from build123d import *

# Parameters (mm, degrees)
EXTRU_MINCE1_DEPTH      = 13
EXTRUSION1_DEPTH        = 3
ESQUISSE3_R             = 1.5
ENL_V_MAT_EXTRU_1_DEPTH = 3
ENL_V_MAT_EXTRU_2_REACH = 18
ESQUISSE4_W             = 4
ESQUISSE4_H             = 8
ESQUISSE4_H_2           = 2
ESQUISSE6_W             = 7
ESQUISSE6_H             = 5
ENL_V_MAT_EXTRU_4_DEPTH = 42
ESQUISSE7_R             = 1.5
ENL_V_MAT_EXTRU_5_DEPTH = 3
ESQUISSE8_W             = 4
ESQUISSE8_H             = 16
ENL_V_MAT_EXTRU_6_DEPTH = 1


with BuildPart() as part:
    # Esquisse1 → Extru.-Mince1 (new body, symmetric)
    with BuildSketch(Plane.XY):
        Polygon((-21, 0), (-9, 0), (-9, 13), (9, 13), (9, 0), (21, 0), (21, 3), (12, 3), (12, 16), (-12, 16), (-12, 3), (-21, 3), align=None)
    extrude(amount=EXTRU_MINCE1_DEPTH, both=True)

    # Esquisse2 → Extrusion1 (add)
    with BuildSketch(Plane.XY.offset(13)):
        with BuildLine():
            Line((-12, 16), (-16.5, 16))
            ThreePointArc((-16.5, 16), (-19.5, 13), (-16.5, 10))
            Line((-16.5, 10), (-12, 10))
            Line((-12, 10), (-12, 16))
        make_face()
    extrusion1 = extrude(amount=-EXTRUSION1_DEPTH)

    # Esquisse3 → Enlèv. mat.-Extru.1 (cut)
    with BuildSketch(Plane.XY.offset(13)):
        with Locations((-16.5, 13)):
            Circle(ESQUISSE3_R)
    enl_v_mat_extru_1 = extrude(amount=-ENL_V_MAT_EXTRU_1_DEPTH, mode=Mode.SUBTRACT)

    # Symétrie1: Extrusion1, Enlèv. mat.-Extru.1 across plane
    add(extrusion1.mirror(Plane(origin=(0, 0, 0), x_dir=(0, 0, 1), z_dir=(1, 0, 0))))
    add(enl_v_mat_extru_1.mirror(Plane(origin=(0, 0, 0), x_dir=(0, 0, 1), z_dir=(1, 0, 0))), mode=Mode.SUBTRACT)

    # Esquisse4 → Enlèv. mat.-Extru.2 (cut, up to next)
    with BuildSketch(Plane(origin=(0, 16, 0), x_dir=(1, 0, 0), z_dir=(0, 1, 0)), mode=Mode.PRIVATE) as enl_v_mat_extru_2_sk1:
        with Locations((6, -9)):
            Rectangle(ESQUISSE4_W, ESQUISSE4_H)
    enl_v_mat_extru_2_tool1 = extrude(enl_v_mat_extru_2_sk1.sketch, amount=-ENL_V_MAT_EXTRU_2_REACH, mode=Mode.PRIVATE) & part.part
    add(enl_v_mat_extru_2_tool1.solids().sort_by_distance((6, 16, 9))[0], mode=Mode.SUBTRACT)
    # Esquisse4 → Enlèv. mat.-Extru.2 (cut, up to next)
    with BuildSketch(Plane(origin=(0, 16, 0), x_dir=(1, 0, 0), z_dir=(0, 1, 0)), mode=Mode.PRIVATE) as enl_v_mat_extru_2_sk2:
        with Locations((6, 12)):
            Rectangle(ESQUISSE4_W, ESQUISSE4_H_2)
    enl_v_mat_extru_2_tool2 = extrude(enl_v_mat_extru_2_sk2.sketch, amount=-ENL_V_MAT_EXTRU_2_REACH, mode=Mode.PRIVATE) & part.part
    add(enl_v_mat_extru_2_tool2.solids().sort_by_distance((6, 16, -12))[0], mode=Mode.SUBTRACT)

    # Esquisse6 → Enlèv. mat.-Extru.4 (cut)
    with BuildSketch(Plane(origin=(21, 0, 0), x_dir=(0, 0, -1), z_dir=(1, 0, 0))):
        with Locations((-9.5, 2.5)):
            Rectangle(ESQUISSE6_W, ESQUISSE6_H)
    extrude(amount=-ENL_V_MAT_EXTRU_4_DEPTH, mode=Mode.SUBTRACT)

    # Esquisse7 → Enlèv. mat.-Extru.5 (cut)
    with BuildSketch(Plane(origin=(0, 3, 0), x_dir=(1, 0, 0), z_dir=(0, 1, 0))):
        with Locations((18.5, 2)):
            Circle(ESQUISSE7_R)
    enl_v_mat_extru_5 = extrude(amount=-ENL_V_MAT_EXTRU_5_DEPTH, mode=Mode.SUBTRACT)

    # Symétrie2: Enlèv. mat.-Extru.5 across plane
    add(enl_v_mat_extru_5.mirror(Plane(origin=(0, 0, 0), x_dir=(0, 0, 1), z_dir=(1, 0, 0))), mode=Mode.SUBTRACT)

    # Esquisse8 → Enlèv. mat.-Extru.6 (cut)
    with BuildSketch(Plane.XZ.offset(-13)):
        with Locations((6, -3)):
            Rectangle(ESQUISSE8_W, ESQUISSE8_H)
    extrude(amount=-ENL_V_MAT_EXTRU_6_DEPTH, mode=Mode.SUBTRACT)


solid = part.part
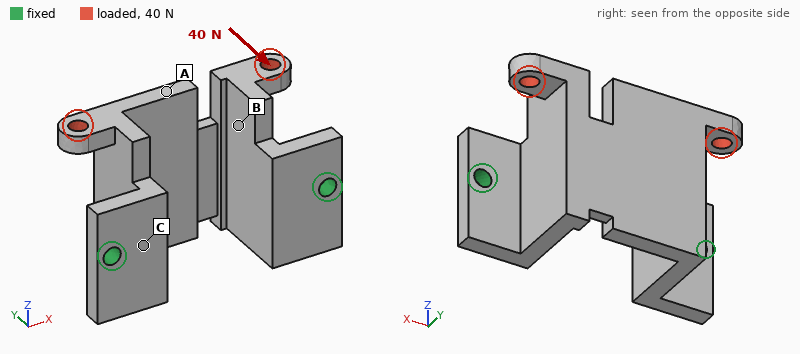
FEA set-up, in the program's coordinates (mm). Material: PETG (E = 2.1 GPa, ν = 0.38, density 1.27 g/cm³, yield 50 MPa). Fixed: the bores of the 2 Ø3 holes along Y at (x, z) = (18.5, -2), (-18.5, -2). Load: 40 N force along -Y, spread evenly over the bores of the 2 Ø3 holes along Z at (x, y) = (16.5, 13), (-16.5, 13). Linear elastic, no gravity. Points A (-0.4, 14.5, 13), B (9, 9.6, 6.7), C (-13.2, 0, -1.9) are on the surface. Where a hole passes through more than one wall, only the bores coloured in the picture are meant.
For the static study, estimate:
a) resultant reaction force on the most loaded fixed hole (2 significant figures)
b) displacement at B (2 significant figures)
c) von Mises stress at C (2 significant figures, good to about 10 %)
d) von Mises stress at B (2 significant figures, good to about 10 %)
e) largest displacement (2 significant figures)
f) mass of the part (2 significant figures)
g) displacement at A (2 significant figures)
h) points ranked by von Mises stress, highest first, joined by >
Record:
21 N
0.21 mm
6.5 MPa
3.8 MPa
0.52 mm
6.0 g
0.33 mm
C > B > A
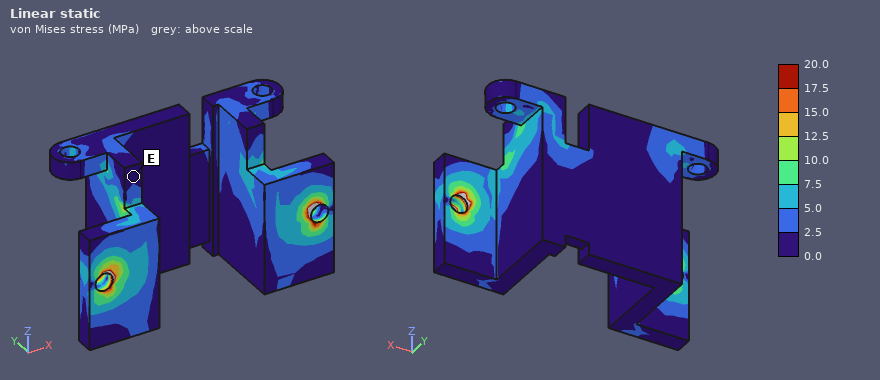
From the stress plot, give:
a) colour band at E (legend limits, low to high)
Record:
0.0 to 2.5 MPa
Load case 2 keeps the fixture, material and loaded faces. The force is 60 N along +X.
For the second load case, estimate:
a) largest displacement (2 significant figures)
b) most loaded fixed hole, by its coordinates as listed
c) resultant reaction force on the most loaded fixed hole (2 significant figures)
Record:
0.58 mm
(-18.5, -2)
42 N
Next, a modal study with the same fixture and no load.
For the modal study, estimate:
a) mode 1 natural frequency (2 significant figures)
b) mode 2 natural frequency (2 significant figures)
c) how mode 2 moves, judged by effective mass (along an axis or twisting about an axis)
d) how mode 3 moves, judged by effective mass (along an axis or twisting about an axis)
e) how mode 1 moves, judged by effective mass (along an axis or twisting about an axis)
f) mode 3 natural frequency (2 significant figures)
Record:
960 Hz
1500 Hz
along X
along X
along Z
2000 Hz
